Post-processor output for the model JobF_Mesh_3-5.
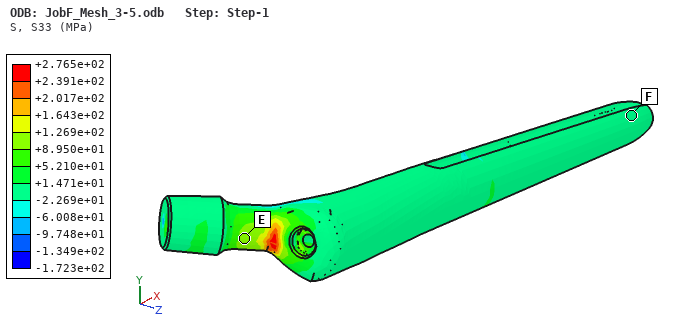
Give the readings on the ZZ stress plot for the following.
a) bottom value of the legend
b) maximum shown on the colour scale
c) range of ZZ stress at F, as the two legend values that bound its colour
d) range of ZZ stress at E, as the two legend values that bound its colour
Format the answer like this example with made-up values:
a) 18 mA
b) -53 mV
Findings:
a) -1.723e+02 MPa
b) +2.765e+02 MPa
c) -2.269e+01 to +1.471e+01 MPa
d) +8.950e+01 to +1.269e+02 MPa
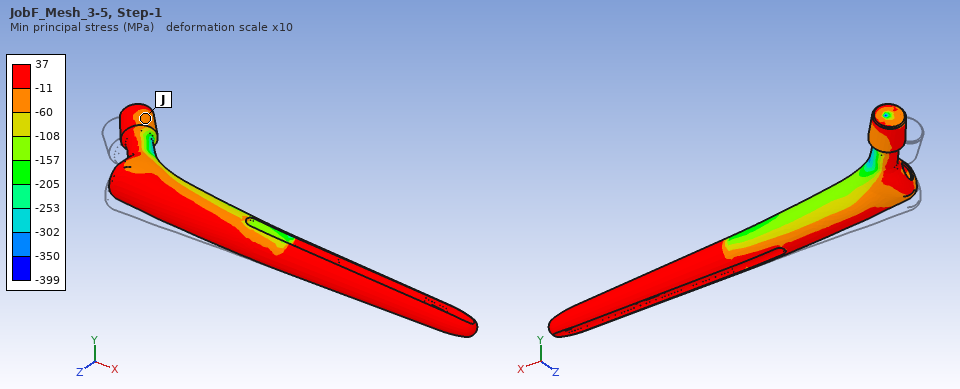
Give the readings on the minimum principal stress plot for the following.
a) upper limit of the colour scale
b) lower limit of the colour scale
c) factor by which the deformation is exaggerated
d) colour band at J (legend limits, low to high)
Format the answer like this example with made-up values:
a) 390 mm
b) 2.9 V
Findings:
a) 37 MPa
b) -399 MPa
c) 10
d) -60 to -11 MPa
